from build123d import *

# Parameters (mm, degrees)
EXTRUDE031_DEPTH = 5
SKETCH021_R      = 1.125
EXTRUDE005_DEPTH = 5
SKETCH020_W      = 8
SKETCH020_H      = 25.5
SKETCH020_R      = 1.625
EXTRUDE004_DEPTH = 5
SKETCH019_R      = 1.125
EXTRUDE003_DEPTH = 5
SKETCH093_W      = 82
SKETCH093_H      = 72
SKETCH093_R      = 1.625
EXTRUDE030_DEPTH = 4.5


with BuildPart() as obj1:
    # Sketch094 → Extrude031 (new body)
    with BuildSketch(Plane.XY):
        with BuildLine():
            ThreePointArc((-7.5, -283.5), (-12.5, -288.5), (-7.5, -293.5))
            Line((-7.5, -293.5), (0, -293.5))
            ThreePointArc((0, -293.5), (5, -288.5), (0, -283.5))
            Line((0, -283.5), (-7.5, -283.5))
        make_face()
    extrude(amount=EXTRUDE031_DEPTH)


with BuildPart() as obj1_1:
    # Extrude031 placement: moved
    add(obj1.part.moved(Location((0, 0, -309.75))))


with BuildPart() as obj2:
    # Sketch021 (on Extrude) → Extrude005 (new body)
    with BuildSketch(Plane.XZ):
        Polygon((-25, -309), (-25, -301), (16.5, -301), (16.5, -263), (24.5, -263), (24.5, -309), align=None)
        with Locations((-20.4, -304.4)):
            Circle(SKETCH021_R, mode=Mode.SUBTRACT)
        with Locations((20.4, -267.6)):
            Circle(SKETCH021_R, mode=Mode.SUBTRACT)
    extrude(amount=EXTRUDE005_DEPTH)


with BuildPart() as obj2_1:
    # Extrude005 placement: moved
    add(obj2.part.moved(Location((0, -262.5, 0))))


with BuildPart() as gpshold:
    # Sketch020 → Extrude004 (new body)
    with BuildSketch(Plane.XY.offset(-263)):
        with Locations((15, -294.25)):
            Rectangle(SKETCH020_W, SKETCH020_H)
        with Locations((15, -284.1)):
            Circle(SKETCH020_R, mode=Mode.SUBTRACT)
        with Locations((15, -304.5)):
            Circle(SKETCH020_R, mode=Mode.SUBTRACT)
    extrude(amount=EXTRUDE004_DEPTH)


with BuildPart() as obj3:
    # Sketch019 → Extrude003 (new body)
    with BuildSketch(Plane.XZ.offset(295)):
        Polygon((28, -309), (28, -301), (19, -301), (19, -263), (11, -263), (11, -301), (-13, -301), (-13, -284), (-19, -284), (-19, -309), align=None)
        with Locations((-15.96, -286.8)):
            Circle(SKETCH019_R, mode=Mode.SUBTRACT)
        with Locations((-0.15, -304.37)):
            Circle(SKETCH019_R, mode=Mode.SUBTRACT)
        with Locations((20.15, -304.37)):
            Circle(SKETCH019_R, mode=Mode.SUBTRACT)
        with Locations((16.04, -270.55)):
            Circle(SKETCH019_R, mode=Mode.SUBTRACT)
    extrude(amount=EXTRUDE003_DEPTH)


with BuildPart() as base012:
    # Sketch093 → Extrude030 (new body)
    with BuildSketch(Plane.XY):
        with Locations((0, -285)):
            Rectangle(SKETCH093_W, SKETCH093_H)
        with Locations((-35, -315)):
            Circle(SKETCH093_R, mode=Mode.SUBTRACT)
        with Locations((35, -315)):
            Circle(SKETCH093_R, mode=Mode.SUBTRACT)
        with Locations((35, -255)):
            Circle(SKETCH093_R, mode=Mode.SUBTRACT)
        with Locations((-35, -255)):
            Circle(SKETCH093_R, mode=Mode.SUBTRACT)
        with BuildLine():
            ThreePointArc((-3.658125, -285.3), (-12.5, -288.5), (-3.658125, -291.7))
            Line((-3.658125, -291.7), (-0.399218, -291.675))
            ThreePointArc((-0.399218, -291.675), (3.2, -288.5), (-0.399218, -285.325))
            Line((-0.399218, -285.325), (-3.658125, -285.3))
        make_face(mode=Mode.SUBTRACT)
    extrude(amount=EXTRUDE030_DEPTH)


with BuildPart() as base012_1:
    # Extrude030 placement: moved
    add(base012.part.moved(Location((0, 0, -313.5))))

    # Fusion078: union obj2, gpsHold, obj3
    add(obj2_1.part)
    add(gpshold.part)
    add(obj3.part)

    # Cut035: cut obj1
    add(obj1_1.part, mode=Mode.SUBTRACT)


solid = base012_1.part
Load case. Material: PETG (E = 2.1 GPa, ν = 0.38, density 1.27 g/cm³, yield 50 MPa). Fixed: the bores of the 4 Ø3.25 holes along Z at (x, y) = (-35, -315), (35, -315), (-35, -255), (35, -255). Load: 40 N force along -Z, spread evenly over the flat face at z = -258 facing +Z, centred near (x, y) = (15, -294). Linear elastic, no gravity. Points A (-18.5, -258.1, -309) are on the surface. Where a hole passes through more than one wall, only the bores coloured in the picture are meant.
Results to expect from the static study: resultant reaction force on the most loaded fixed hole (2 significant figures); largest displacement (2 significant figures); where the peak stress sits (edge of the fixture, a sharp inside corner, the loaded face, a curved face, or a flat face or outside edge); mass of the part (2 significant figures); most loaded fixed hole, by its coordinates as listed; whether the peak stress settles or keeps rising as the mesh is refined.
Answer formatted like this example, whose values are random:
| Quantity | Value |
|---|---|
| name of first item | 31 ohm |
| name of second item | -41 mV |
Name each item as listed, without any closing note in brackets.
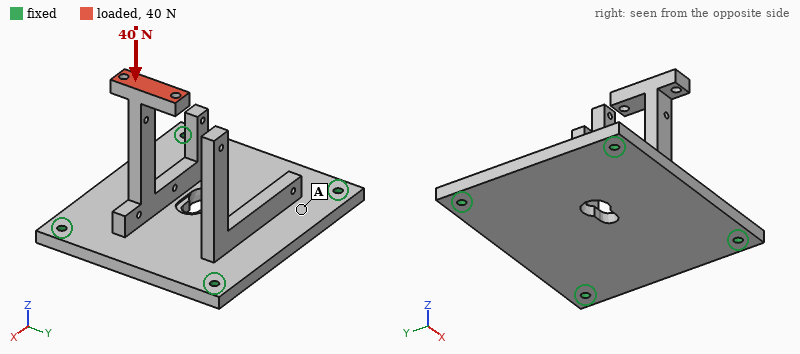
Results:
| Quantity | Value |
|---|---|
| resultant reaction force on the most loaded fixed hole | 21 N |
| largest displacement | 1.2 mm |
| where the peak stress sits | a sharp inside corner |
| mass of the part | 43 g |
| most loaded fixed hole, by its coordinates as listed | (35, -315) |
| whether the peak stress settles or keeps rising as the mesh is refined | keeps rising |
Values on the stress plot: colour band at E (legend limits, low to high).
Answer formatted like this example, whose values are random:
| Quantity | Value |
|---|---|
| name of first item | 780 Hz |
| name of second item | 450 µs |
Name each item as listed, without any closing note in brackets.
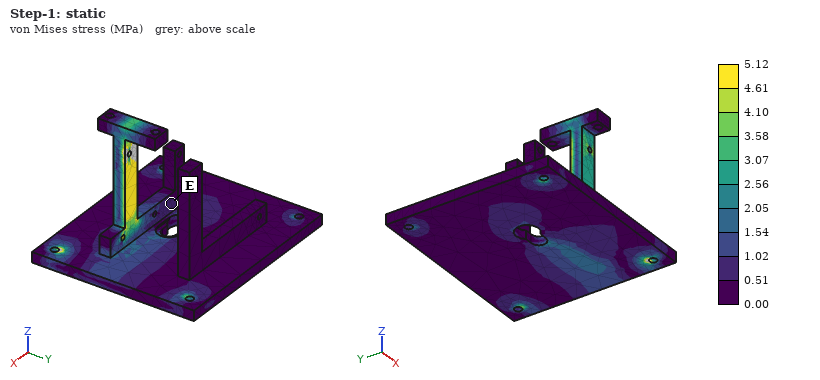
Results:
| Quantity | Value |
|---|---|
| colour band at E | 0.51 to 1.02 MPa |
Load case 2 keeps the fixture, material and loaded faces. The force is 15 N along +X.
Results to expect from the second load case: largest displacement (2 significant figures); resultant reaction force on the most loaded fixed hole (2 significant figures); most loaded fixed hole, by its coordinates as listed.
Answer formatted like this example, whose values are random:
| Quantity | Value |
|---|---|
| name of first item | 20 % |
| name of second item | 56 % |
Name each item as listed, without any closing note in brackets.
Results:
| Quantity | Value |
|---|---|
| largest displacement | 1.5 mm |
| resultant reaction force on the most loaded fixed hole | 13 N |
| most loaded fixed hole, by its coordinates as listed | (-35, -315) |
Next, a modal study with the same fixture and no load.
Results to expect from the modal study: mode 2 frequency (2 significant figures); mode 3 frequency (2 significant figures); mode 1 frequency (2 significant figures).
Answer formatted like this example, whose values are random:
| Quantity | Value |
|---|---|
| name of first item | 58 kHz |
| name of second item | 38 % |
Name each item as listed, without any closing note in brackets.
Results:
| Quantity | Value |
|---|---|
| mode 2 frequency | 460 Hz |
| mode 3 frequency | 490 Hz |
| mode 1 frequency | 270 Hz |
